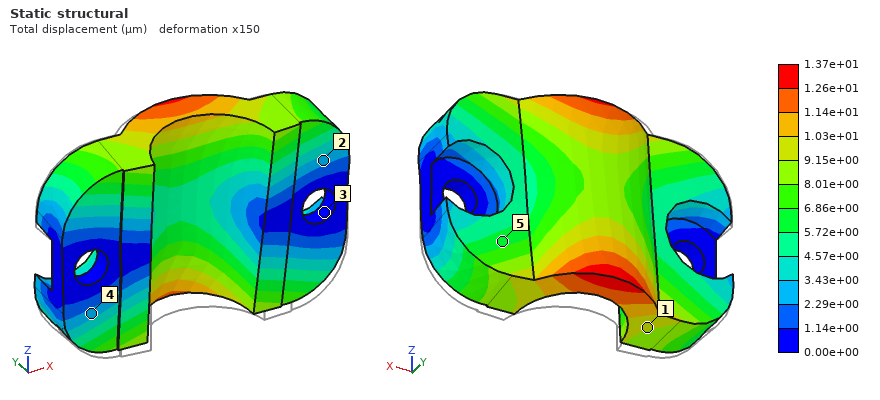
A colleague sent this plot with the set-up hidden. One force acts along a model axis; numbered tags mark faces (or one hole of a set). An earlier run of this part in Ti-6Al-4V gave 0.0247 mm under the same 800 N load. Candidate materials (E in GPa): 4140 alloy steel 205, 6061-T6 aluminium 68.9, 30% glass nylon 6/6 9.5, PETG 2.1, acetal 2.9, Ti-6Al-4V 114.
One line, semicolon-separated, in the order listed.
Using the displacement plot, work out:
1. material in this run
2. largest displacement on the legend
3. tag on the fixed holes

4140 alloy steel; 1.37e+01 µm; 3
